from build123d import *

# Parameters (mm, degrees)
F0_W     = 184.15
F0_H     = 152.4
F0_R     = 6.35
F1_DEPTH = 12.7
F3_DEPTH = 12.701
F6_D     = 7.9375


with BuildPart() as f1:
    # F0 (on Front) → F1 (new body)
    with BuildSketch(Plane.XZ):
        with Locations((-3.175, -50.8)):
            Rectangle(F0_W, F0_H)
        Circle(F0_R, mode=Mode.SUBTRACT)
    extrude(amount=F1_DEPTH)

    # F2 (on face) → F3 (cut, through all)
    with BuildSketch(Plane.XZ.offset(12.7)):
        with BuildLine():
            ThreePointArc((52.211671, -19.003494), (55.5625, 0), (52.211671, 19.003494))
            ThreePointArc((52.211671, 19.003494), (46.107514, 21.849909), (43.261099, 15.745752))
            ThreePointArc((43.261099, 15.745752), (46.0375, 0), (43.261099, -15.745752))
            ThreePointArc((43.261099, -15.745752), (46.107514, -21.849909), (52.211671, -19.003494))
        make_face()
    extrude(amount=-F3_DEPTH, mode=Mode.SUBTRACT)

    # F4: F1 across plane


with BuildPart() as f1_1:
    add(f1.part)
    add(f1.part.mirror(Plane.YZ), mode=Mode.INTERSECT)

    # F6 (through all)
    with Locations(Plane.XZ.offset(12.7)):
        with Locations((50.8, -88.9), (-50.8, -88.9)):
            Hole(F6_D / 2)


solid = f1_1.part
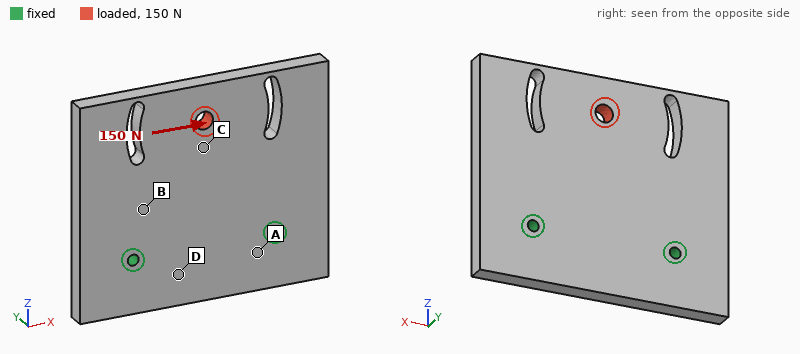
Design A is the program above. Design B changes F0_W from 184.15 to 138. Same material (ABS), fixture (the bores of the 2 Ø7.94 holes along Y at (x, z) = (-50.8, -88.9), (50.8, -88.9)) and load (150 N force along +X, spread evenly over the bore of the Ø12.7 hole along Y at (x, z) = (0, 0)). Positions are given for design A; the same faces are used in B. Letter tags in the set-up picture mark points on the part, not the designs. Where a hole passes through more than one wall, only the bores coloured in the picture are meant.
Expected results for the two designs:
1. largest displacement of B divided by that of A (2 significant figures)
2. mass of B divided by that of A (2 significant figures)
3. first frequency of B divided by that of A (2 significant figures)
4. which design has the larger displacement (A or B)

1.2
0.73
1.0
B
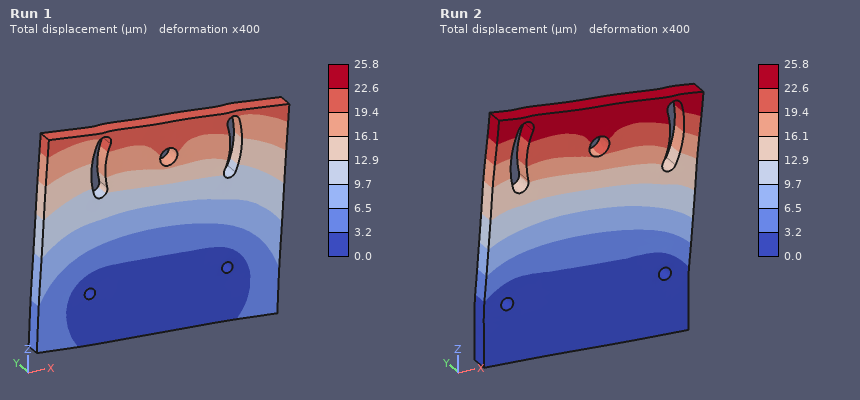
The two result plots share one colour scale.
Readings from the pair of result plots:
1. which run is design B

Run 2
